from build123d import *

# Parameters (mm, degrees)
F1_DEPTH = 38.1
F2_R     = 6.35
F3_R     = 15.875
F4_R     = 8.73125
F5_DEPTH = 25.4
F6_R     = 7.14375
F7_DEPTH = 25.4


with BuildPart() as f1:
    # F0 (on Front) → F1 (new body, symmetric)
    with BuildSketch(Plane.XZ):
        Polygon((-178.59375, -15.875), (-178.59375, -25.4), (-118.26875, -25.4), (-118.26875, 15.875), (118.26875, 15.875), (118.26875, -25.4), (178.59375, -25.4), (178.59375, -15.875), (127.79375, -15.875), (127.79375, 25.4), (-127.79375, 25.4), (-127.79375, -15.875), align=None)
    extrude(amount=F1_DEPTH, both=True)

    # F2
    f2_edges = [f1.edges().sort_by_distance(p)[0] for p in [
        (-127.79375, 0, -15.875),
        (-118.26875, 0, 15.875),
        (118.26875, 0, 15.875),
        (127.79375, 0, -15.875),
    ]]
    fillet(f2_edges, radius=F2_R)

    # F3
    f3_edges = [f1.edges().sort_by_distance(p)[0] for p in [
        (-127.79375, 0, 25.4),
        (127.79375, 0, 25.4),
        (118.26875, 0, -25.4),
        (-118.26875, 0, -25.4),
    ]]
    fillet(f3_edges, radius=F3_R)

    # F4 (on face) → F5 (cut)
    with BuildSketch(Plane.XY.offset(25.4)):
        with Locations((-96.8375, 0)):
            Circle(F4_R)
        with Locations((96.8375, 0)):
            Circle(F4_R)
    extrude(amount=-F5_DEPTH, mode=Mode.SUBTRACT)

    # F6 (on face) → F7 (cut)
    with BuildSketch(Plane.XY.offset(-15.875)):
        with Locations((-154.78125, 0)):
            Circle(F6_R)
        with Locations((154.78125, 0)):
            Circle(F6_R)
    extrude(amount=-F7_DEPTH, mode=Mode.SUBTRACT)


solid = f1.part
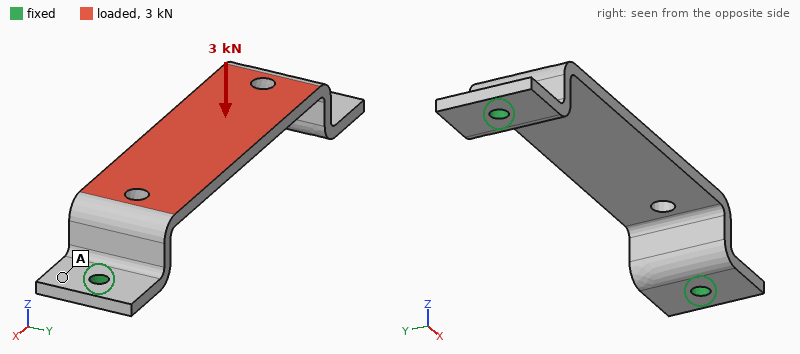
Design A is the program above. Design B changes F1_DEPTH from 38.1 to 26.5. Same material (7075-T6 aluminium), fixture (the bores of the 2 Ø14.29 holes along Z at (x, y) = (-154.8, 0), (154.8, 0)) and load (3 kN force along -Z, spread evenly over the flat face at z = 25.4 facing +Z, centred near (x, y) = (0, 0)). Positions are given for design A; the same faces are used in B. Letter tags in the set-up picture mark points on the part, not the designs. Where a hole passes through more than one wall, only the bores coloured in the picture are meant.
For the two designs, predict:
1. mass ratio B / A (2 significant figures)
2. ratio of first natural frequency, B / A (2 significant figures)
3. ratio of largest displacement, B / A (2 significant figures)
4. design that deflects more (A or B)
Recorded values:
0.69
0.99
1.5
B
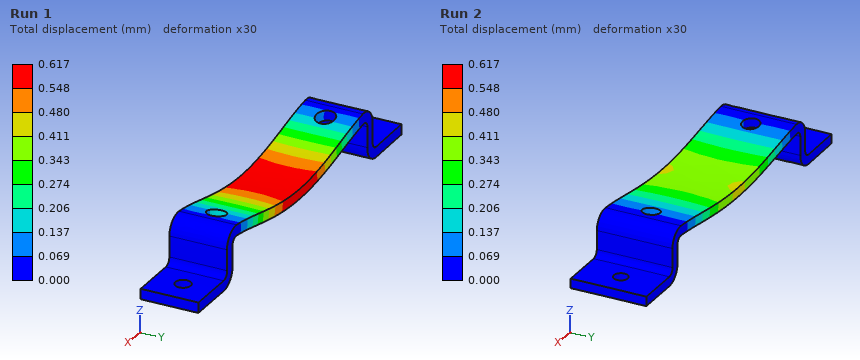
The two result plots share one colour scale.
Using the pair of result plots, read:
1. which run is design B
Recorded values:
Run 1
